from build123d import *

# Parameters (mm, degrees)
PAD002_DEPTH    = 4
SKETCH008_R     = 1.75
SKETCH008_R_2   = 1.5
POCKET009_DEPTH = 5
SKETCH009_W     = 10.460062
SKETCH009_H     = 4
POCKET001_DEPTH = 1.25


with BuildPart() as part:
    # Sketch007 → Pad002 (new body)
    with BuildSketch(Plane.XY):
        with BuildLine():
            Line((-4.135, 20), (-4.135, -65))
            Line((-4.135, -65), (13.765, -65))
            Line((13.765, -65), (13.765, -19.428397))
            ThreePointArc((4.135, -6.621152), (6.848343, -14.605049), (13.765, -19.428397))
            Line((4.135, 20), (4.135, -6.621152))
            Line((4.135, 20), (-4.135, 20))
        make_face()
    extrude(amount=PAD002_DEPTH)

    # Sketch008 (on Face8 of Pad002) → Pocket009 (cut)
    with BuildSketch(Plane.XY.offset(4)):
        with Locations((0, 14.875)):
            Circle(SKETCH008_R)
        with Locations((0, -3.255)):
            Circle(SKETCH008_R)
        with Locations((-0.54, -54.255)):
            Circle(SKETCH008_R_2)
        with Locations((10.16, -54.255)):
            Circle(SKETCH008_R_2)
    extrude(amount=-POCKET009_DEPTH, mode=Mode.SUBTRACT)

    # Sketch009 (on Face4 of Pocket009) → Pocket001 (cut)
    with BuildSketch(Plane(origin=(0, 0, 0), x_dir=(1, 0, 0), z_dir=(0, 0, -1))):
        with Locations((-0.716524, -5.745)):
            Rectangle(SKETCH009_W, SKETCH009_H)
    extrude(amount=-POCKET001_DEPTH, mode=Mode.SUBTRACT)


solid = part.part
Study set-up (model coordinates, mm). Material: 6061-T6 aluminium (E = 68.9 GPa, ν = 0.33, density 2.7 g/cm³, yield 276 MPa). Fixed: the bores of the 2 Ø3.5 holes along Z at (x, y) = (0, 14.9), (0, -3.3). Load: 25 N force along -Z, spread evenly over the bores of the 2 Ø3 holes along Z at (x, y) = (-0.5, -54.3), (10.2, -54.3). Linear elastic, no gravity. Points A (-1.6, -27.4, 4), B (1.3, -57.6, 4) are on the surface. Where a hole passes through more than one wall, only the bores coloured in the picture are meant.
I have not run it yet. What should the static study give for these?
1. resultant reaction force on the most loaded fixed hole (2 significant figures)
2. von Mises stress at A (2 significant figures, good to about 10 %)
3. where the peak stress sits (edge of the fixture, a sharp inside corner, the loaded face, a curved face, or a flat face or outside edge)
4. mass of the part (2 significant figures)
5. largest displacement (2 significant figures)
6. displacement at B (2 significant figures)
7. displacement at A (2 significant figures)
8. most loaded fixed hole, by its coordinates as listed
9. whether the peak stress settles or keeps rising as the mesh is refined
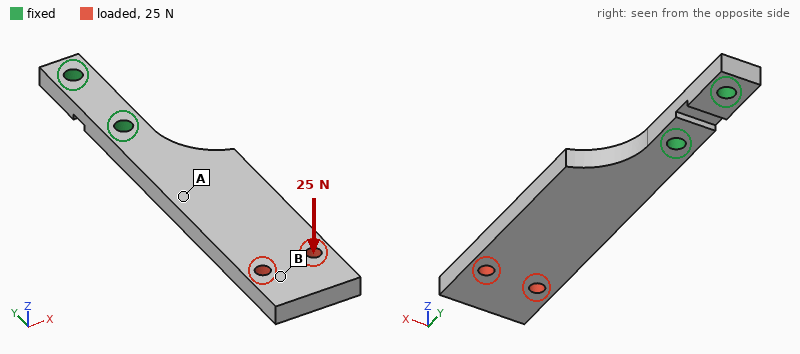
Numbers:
28 N
16 MPa
edge of the fixture
12 g
0.35 mm
0.29 mm
0.082 mm
(0, -3.3)
keeps rising
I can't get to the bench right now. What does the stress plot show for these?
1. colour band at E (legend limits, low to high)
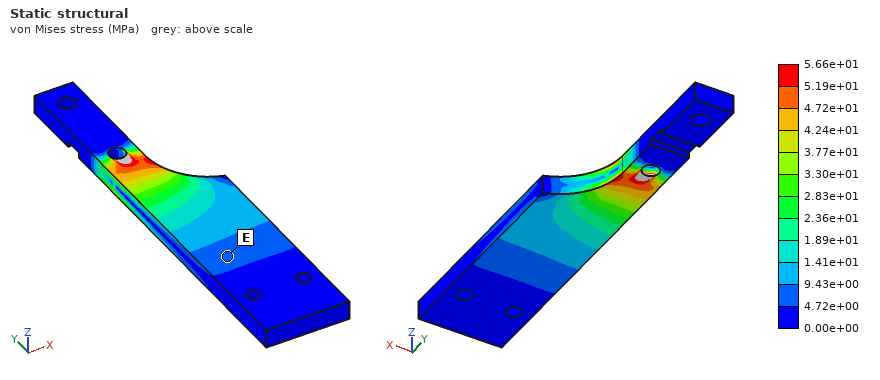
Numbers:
4.72e+00 to 9.43e+00 MPa
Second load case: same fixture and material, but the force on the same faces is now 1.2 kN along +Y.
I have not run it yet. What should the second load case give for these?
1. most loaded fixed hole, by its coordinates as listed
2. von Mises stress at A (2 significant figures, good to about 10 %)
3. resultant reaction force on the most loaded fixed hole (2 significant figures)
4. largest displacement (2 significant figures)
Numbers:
(0, -3.3)
16 MPa
1.2 kN
0.33 mm
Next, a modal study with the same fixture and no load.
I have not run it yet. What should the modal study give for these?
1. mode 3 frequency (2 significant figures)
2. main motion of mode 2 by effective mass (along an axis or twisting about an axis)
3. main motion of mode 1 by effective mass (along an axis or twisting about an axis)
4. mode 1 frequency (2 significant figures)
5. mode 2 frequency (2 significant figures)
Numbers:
3900 Hz
along X
along Z
680 Hz
1400 Hz
